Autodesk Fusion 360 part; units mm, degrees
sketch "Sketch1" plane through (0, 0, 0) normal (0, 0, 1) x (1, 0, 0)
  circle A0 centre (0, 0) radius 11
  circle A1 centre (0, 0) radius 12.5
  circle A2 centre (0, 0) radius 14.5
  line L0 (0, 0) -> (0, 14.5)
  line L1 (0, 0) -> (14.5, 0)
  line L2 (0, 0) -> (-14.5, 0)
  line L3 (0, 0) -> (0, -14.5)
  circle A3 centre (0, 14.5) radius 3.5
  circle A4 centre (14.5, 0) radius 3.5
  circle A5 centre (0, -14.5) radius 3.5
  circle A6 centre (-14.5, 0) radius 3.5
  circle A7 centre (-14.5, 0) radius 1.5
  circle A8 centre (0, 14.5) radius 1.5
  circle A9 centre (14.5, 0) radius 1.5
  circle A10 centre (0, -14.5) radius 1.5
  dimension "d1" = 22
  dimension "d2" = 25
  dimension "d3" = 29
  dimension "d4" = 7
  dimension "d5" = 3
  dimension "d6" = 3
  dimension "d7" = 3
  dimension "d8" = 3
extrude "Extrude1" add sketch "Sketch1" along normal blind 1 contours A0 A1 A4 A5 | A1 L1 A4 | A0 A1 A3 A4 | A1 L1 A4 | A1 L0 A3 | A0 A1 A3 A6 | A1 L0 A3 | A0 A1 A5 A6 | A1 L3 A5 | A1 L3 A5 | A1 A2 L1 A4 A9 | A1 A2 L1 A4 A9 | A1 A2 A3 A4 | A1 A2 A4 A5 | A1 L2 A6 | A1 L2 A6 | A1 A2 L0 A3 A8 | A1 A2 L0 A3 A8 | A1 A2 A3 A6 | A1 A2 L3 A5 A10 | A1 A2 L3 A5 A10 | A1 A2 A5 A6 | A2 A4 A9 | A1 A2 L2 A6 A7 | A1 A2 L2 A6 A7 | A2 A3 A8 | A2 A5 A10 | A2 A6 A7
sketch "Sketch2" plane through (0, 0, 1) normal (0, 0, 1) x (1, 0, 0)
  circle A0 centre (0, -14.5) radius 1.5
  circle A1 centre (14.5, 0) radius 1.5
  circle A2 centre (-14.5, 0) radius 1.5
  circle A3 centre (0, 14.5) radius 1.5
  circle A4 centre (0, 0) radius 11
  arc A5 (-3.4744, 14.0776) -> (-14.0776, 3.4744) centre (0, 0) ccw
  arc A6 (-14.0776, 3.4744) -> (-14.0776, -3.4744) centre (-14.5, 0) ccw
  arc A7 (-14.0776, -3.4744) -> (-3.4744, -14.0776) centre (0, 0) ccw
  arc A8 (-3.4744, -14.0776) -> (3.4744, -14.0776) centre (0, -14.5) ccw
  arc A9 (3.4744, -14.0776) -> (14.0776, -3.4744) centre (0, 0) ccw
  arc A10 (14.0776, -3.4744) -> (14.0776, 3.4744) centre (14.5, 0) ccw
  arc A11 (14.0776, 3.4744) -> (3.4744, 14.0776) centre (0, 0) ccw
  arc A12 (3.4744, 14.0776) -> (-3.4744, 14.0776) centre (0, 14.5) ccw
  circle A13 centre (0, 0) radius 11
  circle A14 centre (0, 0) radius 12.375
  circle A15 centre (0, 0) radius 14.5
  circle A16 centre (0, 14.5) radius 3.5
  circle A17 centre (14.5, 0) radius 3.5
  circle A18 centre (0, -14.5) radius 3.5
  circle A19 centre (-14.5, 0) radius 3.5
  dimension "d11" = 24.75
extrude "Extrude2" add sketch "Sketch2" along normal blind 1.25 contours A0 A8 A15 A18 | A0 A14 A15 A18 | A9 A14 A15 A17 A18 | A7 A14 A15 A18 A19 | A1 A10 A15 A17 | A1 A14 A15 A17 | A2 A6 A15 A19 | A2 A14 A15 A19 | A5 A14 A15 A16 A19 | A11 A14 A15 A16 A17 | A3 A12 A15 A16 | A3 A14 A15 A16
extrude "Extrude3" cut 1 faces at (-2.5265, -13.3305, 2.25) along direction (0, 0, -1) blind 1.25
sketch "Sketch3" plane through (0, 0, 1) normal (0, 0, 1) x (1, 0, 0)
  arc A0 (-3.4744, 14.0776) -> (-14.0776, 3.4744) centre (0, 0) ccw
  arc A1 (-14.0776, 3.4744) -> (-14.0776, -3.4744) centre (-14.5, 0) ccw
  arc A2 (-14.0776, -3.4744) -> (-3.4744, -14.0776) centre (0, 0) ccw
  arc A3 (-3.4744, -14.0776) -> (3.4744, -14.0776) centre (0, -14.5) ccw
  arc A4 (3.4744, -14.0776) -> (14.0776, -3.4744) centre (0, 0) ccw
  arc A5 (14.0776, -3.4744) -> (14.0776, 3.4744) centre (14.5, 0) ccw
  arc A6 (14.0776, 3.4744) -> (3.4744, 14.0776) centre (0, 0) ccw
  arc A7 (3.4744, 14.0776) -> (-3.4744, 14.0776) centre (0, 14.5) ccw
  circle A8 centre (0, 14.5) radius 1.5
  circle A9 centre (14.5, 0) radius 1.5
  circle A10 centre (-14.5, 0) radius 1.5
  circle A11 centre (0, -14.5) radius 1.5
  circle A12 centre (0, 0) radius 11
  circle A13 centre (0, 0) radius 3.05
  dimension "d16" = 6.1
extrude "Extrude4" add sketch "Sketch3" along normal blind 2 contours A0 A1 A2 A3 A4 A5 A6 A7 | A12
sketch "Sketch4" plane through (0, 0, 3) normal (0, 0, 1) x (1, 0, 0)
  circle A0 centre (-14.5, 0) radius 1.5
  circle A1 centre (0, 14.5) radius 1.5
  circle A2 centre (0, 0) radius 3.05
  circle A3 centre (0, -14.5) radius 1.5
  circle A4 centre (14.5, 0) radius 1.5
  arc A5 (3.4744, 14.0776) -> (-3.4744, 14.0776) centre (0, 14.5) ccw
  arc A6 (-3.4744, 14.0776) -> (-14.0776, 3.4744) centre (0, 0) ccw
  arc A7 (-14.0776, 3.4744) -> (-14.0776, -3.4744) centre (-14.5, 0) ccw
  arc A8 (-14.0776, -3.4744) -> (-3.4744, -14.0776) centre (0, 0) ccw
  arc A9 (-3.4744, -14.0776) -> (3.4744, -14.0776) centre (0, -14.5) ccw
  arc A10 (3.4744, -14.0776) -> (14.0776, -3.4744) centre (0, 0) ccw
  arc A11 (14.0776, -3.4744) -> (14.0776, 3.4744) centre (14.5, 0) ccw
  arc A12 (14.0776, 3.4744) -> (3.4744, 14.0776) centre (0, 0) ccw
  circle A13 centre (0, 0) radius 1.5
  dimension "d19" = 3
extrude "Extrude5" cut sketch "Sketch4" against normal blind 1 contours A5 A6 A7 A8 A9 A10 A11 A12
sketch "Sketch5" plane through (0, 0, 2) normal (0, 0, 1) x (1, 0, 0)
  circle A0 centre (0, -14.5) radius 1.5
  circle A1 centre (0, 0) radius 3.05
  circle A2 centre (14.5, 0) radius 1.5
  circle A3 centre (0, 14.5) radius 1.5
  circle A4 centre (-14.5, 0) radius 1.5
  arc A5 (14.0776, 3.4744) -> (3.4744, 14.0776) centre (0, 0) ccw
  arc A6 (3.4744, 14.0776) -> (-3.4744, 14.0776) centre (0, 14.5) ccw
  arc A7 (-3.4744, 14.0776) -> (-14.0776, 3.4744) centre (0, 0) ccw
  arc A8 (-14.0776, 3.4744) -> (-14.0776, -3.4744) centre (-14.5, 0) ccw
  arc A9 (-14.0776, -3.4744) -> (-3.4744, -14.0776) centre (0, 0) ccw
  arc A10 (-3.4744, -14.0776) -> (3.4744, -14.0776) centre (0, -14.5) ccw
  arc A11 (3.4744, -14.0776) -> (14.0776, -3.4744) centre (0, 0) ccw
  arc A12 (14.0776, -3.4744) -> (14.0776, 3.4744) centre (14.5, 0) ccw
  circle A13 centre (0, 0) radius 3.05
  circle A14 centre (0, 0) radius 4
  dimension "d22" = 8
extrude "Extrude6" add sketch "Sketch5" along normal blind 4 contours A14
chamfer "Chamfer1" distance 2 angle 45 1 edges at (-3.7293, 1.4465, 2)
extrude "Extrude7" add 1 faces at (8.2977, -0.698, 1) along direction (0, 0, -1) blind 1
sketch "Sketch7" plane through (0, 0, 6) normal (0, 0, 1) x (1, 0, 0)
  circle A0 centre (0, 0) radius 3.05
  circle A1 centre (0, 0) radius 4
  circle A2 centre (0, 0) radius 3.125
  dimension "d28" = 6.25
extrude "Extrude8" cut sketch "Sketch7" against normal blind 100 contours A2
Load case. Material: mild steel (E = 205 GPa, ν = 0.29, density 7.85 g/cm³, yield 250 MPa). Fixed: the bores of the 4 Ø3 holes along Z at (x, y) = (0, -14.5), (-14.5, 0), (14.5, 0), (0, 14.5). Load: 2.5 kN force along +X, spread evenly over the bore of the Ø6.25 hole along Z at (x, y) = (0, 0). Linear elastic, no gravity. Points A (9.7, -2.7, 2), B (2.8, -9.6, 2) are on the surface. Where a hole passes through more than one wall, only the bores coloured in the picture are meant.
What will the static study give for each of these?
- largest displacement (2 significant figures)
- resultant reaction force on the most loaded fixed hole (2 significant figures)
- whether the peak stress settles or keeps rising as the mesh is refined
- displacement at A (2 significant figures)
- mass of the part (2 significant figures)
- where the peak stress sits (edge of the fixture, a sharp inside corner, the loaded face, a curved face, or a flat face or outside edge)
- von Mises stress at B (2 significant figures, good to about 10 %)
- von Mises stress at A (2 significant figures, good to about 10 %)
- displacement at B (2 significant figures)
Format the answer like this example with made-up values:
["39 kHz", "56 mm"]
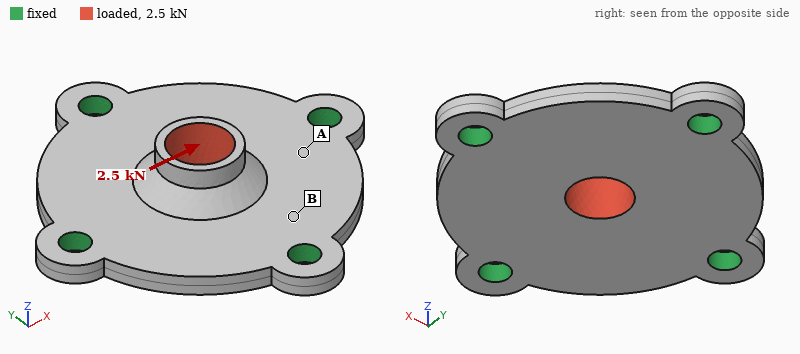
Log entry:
["12 µm", "920 N", "keeps rising", "3.2 µm", "12 g", "edge of the fixture", "33 MPa", "70 MPa", "2.2 µm"]
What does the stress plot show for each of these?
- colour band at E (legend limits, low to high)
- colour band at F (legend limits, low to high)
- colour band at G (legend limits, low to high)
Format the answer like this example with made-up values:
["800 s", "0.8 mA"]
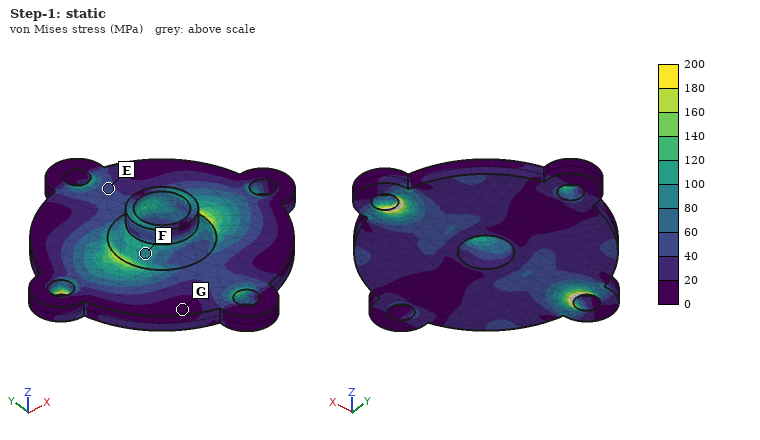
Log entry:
["40 to 60 MPa", "80 to 100 MPa", "0 to 20 MPa"]
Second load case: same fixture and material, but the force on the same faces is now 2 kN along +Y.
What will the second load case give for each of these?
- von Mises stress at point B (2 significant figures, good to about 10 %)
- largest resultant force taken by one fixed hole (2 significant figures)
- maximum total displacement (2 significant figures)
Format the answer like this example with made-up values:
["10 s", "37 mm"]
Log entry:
["56 MPa", "740 N", "9.6 µm"]
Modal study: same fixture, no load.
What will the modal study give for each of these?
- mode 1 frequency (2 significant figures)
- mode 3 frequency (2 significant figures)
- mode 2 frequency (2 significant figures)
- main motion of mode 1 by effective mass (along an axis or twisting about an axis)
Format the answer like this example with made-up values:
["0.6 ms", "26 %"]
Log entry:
["20 kHz", "28 kHz", "28 kHz", "along Z"]
